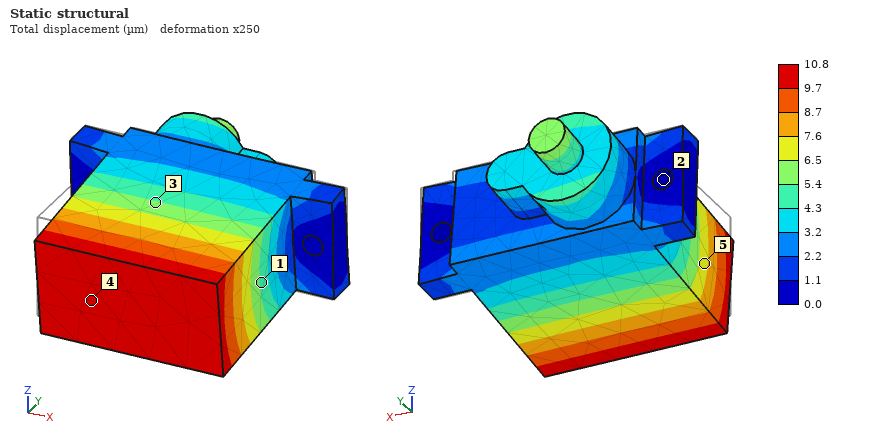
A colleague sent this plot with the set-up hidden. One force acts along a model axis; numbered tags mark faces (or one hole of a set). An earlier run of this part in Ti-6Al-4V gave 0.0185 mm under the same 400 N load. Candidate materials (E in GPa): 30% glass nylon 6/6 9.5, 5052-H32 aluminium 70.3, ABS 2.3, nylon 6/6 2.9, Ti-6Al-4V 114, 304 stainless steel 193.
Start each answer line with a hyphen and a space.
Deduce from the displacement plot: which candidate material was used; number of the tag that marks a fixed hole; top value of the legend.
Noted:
- 304 stainless steel
- 2
- 10.8 µm
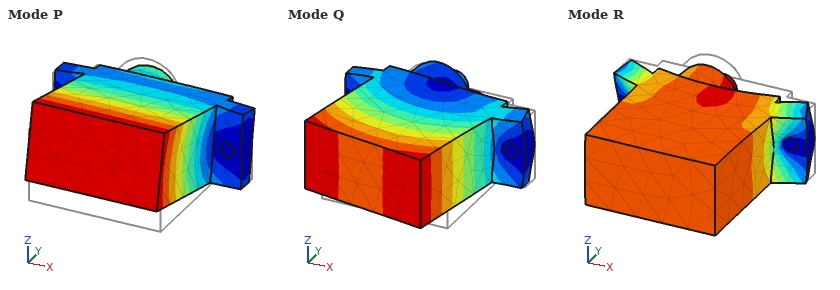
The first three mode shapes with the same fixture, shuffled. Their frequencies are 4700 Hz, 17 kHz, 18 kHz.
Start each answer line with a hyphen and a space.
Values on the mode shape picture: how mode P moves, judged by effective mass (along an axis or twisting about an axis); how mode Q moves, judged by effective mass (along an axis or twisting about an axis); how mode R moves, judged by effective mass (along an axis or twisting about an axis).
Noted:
- along Z
- along X
- along Y
